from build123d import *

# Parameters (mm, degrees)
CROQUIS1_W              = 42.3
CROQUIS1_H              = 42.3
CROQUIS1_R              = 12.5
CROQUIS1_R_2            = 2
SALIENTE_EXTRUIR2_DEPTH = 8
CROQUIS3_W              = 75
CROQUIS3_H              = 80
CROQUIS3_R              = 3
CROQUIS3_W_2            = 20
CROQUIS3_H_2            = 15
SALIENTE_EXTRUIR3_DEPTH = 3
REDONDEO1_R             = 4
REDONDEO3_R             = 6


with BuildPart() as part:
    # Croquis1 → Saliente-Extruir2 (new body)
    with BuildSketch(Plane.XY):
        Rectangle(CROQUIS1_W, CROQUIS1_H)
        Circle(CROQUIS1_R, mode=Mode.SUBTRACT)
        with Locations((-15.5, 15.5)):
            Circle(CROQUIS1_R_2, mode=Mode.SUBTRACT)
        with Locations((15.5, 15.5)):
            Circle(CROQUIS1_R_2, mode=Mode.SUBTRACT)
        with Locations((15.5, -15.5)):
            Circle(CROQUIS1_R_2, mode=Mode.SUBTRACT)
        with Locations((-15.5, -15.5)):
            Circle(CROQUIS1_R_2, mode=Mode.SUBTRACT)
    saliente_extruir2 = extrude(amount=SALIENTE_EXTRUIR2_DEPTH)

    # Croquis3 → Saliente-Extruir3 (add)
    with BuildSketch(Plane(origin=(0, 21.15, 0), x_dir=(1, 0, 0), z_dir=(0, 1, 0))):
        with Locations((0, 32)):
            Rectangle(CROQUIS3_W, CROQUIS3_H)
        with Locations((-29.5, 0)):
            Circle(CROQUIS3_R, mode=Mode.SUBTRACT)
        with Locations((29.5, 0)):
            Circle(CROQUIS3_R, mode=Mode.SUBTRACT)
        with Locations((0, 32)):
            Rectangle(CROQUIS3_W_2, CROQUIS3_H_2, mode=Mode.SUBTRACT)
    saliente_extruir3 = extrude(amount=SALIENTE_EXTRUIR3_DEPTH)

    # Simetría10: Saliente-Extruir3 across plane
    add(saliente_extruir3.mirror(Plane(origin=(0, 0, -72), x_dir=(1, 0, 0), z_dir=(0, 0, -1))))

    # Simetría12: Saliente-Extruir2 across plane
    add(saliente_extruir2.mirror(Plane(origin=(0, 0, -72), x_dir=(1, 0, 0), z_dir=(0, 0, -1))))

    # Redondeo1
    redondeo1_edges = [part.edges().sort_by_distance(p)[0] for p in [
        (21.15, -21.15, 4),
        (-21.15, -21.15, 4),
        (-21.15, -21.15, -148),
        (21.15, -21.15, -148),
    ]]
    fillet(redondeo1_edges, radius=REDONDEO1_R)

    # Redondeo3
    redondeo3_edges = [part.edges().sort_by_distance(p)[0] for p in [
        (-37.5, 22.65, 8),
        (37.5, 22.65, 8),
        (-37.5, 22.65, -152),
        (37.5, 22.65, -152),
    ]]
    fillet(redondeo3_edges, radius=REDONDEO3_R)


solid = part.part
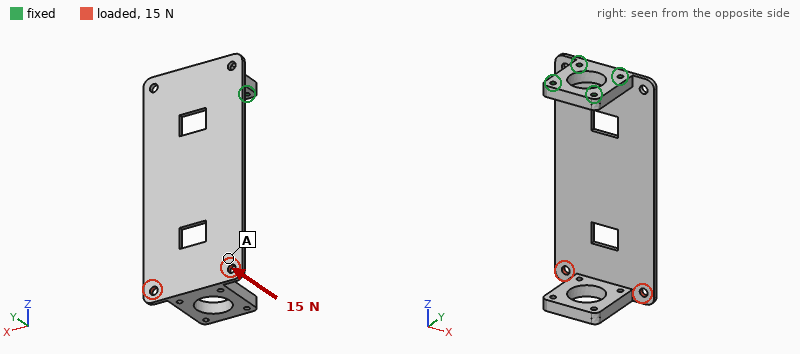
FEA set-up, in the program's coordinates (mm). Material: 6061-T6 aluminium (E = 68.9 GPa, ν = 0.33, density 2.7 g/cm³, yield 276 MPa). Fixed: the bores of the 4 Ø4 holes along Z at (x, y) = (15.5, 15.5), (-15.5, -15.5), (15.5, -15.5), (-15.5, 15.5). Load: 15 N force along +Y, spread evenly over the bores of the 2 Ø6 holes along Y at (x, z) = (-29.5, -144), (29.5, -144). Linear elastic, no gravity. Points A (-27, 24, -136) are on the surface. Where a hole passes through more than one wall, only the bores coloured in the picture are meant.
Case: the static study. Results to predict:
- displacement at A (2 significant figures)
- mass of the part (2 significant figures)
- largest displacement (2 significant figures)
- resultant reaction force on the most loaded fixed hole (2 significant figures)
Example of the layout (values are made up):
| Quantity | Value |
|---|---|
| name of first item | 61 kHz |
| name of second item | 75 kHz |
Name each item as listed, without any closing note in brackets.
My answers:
| Quantity | Value |
|---|---|
| displacement at A | 1.4 mm |
| mass of the part | 140 g |
| largest displacement | 1.8 mm |
| resultant reaction force on the most loaded fixed hole | 27 N |
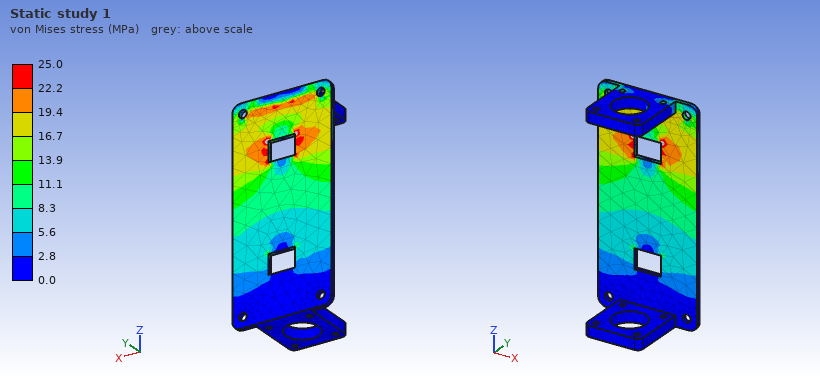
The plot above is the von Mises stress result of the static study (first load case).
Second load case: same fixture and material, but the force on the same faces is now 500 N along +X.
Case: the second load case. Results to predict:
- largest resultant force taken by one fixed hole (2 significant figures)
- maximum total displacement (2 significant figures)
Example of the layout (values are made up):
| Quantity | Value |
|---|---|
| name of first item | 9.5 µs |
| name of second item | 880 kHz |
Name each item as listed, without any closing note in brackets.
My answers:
| Quantity | Value |
|---|---|
| largest resultant force taken by one fixed hole | 2.2 kN |
| maximum total displacement | 0.34 mm |
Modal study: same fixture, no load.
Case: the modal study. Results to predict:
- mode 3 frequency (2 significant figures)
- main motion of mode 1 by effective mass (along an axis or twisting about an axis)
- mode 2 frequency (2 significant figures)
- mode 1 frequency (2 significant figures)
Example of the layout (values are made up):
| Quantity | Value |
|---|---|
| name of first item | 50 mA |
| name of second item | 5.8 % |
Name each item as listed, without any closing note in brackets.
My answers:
| Quantity | Value |
|---|---|
| mode 3 frequency | 410 Hz |
| main motion of mode 1 by effective mass | along Y |
| mode 2 frequency | 280 Hz |
| mode 1 frequency | 67 Hz |
